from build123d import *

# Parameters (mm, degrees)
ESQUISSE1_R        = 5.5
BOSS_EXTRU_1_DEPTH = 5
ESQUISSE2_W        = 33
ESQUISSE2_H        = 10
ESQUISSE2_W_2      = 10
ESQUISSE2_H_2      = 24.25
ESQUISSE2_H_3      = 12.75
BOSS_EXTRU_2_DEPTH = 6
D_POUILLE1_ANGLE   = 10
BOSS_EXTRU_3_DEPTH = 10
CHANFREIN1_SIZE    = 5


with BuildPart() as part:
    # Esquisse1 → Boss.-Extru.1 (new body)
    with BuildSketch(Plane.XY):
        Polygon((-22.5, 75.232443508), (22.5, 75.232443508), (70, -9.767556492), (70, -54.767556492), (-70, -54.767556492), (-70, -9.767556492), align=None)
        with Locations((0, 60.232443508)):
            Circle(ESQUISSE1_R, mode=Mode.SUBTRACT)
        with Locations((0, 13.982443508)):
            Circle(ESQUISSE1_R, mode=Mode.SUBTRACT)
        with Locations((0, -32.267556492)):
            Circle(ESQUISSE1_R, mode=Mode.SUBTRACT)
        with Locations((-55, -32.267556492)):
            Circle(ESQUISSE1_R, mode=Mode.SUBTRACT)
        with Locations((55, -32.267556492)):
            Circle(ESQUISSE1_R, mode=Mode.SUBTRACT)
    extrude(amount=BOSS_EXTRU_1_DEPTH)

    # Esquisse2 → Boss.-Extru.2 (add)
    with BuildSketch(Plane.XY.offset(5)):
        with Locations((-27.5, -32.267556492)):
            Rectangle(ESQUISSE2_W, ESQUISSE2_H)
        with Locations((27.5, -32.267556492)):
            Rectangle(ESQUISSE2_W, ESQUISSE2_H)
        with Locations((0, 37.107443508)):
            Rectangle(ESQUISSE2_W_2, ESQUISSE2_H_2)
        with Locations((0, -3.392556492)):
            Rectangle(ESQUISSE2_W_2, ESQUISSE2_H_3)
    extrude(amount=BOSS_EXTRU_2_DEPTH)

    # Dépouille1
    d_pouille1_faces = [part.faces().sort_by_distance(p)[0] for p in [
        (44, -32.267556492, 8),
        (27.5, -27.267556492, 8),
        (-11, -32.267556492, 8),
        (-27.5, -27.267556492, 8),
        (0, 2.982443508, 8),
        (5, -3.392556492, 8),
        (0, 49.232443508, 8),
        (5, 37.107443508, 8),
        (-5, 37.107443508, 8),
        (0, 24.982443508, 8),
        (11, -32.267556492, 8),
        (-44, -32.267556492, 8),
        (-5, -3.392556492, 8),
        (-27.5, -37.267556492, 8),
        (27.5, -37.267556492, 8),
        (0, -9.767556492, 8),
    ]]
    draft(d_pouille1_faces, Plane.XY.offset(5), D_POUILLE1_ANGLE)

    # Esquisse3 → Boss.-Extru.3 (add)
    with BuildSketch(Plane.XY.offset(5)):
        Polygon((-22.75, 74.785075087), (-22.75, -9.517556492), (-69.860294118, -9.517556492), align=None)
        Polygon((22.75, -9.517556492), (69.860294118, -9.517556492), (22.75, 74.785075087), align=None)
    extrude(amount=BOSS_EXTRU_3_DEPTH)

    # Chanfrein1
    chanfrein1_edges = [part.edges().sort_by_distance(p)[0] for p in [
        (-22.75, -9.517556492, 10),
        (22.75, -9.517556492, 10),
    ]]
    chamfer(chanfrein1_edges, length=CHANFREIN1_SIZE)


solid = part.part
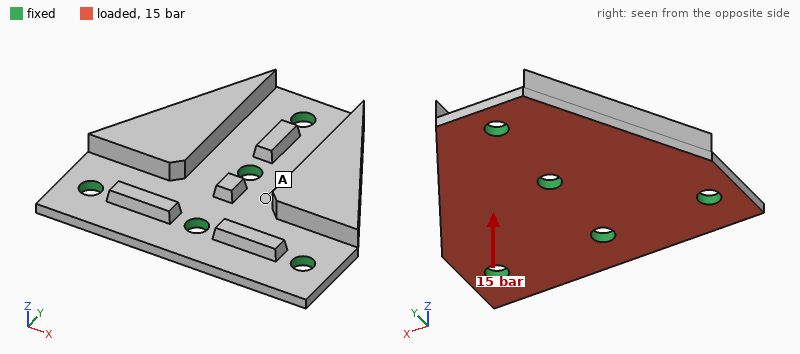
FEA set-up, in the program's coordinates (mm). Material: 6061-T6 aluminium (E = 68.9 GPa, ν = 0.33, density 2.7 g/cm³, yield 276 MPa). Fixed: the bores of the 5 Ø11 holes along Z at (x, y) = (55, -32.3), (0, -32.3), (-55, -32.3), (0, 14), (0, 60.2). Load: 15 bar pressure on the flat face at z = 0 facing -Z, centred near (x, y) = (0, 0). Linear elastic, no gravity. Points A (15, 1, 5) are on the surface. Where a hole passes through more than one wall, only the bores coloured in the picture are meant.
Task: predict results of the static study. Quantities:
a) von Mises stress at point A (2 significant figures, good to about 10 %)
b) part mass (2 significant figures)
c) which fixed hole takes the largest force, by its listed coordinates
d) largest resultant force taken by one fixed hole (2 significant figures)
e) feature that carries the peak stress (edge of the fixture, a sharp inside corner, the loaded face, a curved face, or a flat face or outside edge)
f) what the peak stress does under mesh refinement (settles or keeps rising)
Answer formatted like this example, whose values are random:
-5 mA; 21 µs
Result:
35 MPa; 310 g; (0, 60.2); 5.2 kN; edge of the fixture; keeps rising
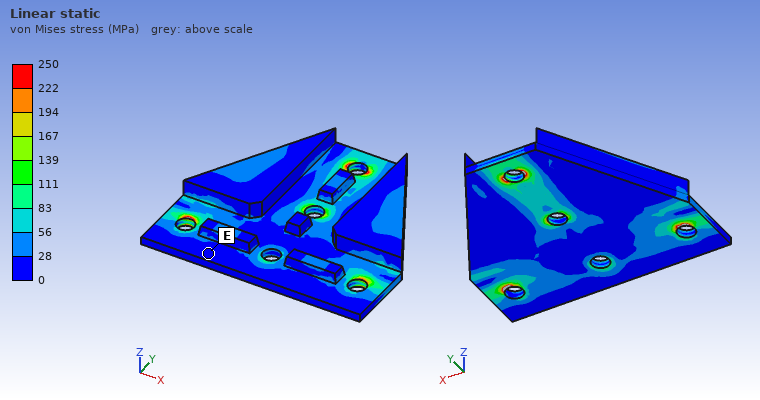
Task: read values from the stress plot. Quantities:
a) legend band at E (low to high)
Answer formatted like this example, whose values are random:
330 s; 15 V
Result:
0 to 28 MPa
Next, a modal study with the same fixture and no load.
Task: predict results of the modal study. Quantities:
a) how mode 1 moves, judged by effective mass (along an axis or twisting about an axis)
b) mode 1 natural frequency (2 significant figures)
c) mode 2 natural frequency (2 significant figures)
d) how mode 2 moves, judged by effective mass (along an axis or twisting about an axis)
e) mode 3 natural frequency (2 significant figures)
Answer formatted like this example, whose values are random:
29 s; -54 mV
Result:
twisting about Y; 2800 Hz; 2900 Hz; along Z; 6300 Hz
